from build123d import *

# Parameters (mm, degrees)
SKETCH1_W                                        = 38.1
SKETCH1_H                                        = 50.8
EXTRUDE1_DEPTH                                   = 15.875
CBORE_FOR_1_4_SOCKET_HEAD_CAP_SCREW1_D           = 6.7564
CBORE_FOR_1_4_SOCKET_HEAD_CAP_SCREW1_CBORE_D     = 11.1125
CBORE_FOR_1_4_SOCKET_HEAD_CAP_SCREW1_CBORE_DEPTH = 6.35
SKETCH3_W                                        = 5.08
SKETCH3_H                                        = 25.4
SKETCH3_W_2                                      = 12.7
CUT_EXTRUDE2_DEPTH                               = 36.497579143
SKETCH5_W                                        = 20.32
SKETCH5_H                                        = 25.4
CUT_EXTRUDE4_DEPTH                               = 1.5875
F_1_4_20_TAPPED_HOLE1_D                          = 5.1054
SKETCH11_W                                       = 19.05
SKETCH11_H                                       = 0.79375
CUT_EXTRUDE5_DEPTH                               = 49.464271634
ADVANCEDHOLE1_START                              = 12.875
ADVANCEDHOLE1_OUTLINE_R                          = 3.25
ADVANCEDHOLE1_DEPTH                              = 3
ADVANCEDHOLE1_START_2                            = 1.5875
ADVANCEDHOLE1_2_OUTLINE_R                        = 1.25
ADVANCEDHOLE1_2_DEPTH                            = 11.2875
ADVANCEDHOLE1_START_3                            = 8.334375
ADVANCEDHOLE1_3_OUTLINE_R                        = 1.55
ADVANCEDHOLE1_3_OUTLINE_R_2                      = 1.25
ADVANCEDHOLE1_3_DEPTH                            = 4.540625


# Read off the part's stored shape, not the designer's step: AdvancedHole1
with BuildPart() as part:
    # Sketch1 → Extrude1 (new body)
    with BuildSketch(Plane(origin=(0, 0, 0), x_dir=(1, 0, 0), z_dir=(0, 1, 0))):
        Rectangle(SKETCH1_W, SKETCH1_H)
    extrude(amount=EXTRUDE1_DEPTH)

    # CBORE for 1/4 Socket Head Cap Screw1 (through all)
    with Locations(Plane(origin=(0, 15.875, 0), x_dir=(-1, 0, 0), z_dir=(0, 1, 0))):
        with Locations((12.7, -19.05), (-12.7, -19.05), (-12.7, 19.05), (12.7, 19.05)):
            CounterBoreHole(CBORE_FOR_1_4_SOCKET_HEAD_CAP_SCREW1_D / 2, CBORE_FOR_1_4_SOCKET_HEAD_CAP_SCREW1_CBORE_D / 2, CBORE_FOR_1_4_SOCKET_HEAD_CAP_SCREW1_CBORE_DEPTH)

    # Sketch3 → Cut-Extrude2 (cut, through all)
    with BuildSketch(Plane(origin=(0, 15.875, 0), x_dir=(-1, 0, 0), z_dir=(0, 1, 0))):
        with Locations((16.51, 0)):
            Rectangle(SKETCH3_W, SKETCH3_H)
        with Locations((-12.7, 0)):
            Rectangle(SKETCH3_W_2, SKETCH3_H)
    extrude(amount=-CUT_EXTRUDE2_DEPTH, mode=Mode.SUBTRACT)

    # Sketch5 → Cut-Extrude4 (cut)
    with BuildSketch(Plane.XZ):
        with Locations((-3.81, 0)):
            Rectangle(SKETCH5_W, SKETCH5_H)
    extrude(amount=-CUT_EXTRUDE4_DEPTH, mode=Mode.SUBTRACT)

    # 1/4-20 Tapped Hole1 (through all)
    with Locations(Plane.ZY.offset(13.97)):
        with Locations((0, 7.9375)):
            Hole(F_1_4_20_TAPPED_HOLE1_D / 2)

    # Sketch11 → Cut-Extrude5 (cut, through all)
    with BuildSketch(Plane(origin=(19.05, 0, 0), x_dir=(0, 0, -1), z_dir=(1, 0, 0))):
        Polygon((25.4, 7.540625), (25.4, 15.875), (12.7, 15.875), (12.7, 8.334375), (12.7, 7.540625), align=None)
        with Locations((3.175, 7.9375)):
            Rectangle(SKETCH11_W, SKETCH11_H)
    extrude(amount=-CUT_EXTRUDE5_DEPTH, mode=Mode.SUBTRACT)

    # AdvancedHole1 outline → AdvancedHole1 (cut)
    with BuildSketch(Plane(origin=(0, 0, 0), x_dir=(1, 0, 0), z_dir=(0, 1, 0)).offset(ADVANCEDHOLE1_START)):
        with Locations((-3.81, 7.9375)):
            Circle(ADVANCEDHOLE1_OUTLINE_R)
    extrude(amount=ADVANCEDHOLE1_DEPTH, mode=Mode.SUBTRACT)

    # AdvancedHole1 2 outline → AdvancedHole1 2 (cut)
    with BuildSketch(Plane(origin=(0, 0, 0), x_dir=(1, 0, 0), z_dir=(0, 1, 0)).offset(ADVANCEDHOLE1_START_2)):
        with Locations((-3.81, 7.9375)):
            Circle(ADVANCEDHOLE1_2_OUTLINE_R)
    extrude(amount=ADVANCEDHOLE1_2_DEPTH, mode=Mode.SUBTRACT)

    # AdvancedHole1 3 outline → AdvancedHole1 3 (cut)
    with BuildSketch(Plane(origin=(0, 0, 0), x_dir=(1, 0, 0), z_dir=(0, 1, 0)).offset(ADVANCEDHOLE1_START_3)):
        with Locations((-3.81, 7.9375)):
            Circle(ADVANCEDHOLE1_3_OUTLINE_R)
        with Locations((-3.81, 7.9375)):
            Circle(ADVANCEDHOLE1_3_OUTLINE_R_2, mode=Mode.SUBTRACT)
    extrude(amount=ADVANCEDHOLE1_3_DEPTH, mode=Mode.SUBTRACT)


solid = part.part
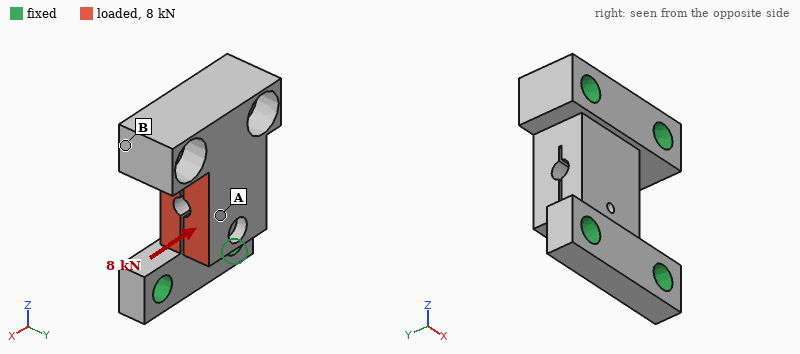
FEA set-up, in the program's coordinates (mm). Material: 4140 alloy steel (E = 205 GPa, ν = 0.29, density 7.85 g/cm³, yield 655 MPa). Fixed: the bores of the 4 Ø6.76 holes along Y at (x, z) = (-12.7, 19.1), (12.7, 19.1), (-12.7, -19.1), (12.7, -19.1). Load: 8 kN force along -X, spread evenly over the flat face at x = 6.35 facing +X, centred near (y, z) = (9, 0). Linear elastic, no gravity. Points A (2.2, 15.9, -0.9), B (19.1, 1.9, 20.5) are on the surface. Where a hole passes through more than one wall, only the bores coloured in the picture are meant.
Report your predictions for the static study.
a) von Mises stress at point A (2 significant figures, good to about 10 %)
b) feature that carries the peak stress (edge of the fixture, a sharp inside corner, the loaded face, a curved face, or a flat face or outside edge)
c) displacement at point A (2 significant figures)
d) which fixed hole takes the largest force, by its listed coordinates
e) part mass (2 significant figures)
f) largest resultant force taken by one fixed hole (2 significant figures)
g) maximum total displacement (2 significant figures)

37 MPa
the loaded face
13 µm
(-12.7, 19.1)
120 g
4.9 kN
27 µm
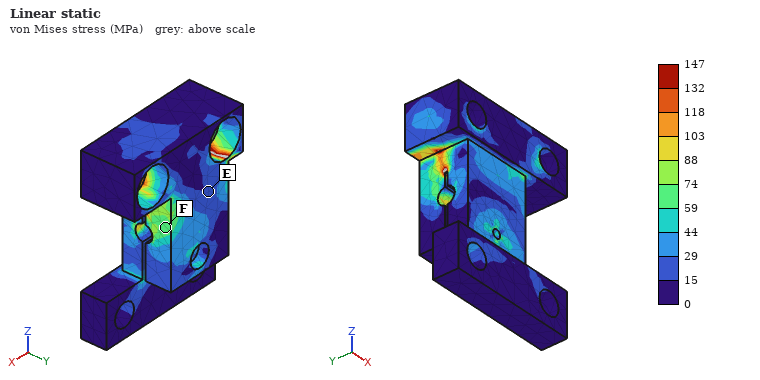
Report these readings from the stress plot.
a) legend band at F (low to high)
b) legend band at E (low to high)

59 to 74 MPa
15 to 29 MPa
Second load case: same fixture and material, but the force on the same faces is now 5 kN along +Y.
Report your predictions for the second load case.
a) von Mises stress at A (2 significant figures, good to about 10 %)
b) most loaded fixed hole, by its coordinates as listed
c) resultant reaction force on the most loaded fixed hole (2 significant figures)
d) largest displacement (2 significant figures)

100 MPa
(12.7, 19.1)
2.9 kN
85 µm
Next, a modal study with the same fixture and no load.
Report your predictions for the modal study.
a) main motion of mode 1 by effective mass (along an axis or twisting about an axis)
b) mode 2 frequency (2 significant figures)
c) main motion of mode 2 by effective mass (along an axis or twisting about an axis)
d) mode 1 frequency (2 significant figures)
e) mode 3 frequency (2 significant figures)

along Y
16 kHz
along X
8400 Hz
21 kHz
